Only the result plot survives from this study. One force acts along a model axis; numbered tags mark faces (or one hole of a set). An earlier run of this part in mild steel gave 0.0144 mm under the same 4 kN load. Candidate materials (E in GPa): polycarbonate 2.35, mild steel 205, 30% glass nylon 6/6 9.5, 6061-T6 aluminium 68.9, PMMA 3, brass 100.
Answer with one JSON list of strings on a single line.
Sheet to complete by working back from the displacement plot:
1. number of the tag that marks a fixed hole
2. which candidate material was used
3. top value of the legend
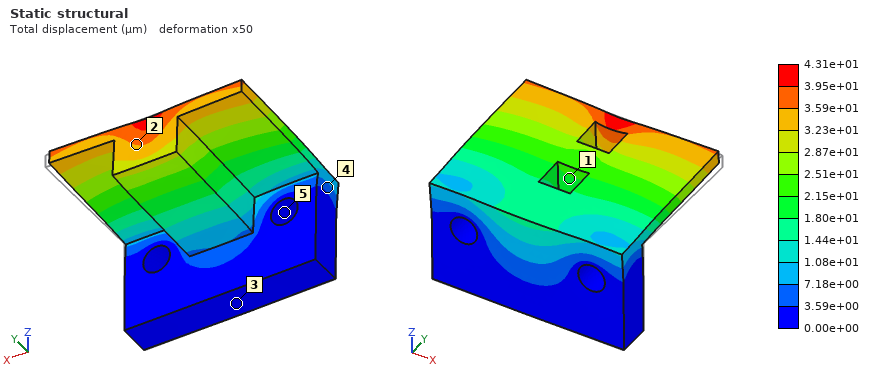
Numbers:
["5", "6061-T6 aluminium", "4.31e+01 µm"]
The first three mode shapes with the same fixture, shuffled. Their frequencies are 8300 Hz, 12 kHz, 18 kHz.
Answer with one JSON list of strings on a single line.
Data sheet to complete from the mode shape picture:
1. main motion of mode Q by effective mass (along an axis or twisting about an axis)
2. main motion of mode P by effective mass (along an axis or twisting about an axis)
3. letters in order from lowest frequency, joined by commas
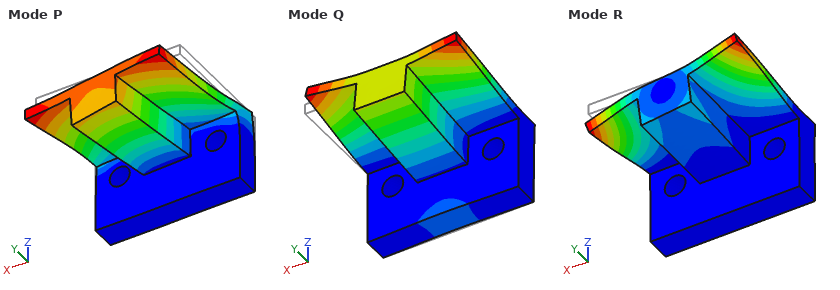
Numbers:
["along Z", "along X", "Q, R, P"]
